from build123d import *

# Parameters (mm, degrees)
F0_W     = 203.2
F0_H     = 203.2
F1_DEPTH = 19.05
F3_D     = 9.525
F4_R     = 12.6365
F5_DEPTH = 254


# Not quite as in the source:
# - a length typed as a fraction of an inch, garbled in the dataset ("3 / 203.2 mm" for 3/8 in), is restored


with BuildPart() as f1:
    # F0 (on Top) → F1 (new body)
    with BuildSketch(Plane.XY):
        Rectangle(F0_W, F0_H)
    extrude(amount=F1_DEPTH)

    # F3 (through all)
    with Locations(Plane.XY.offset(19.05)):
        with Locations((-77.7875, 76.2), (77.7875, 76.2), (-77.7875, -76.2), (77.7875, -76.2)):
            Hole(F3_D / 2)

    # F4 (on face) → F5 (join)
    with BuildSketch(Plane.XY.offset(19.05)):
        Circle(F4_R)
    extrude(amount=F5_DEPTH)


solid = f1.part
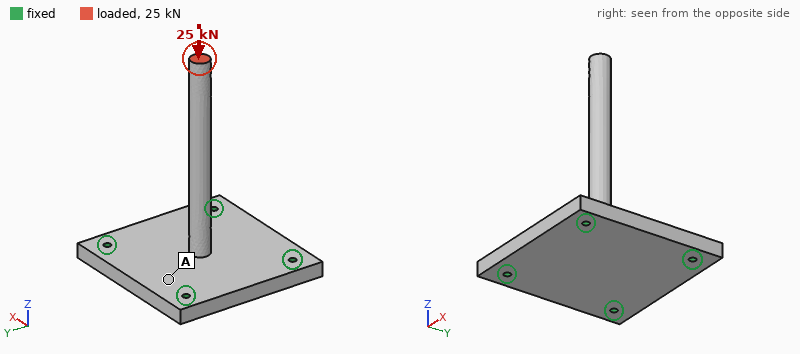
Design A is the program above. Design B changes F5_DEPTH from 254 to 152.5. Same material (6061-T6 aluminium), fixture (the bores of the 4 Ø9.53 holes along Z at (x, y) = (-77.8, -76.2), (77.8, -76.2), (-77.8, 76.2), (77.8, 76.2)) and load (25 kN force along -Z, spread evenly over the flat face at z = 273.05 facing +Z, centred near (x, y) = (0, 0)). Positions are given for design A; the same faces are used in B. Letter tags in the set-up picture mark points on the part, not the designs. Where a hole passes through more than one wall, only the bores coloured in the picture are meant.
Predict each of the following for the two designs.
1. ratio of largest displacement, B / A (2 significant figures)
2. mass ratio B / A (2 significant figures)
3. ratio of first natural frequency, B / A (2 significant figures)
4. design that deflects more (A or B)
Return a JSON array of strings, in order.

["0.81", "0.94", "2.6", "A"]
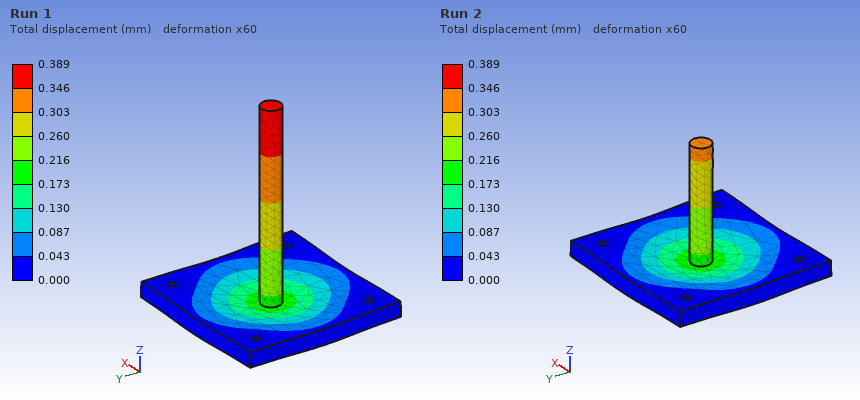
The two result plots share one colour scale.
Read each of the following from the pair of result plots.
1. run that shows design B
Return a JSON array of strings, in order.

["Run 2"]
